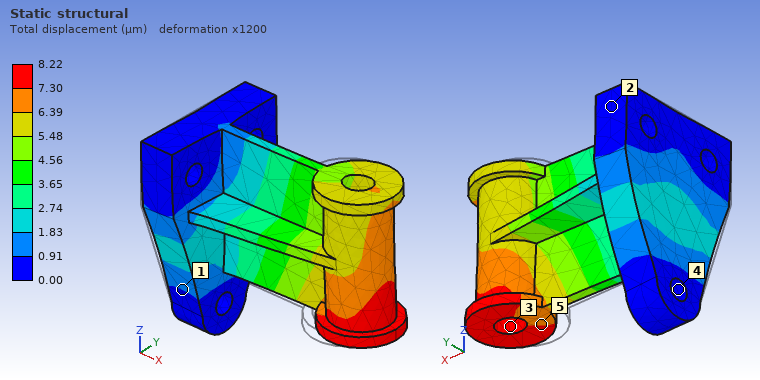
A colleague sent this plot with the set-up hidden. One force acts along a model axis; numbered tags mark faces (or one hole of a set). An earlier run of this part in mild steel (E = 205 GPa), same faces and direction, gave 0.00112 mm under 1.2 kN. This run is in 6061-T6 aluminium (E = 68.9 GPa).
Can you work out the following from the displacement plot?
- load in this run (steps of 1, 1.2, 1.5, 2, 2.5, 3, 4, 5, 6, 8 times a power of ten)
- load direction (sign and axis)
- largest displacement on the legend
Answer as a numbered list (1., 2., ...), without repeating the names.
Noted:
1. 3 kN
2. +X
3. 8.22 µm
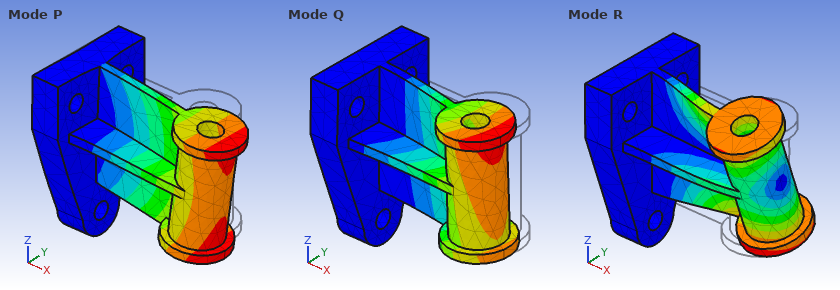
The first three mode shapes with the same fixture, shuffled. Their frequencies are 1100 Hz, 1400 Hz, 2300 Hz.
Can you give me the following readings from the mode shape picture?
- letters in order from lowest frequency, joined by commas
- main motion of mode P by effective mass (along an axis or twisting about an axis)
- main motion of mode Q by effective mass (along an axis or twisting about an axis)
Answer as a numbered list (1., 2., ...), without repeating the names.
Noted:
1. R, Q, P
2. along Z
3. along Y
